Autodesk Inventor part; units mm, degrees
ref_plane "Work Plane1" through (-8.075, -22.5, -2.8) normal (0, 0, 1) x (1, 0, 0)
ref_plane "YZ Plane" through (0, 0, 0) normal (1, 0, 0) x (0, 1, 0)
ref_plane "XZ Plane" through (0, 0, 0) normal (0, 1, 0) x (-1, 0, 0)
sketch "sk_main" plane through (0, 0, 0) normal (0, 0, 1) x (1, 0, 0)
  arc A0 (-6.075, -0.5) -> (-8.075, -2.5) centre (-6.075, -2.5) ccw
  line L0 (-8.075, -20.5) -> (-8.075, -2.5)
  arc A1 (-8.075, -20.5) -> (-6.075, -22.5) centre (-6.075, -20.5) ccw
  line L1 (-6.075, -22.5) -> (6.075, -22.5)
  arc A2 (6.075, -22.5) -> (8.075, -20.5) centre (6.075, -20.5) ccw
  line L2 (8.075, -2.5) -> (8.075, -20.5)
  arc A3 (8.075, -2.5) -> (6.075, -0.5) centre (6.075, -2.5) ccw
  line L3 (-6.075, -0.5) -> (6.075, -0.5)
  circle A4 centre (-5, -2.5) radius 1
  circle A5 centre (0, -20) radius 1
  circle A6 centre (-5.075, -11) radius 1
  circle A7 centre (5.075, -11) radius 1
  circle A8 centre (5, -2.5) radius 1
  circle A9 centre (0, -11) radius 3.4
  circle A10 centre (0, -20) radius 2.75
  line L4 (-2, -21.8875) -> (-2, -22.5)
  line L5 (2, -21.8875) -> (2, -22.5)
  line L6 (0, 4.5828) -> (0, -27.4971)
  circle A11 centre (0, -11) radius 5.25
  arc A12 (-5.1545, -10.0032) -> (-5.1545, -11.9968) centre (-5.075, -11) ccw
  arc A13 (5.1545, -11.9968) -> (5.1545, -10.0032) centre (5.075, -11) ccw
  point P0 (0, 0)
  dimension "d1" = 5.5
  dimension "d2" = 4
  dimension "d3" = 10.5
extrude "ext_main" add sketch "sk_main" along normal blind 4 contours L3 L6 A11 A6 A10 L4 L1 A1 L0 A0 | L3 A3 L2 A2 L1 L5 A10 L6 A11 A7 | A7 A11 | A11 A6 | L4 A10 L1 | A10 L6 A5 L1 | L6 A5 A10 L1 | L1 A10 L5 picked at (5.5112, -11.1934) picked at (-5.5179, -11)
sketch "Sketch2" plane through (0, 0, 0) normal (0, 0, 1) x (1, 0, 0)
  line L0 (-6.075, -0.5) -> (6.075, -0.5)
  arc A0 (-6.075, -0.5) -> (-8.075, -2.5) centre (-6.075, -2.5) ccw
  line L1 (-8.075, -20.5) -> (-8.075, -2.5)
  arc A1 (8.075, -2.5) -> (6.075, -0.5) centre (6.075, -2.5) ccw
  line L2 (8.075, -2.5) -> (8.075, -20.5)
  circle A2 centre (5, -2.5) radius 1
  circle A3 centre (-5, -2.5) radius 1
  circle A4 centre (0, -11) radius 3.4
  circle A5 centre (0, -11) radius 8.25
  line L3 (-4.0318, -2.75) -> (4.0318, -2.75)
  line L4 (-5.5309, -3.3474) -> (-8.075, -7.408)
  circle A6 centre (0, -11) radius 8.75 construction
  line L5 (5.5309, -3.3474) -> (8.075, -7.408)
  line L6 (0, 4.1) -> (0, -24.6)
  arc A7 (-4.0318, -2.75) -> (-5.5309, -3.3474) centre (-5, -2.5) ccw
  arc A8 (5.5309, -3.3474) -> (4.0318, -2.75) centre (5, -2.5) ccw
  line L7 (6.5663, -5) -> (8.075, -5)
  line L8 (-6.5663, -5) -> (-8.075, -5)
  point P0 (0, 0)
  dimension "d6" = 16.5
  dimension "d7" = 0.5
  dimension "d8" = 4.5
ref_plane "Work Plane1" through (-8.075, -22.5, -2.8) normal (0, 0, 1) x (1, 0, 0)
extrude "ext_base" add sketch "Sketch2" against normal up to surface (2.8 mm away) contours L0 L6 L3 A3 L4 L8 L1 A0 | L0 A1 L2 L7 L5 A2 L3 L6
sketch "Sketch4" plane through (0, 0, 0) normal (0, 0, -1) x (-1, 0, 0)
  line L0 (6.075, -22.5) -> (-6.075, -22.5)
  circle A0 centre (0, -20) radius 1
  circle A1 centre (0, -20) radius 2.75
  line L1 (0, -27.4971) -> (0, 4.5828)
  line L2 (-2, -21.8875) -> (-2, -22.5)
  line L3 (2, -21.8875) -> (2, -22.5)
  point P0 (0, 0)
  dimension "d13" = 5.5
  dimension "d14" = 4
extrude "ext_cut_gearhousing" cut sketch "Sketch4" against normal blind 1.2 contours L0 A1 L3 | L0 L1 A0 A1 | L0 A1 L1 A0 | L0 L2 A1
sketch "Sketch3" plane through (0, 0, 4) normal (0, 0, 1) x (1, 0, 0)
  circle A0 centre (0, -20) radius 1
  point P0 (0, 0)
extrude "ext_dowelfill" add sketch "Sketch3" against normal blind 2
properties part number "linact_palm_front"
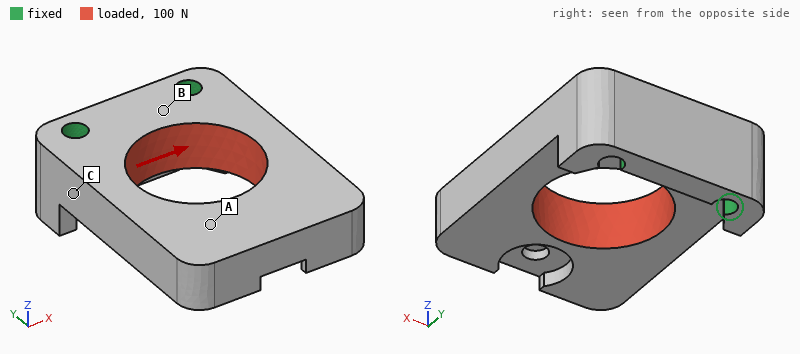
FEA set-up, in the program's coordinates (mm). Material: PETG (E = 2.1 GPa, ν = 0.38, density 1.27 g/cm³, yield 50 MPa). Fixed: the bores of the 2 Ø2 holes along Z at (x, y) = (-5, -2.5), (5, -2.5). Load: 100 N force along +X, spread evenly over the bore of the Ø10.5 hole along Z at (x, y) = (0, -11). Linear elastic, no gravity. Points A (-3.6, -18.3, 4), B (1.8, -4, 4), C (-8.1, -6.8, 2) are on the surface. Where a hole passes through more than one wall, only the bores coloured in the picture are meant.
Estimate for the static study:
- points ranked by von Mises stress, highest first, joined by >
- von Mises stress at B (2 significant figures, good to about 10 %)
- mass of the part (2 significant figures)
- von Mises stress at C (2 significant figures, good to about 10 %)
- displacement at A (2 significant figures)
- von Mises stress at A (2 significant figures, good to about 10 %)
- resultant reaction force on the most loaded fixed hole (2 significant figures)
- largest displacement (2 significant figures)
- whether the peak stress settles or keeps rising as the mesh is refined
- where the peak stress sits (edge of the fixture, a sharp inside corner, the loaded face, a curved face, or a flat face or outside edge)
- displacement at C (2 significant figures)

C > B > A
5.5 MPa
1.4 g
10 MPa
0.15 mm
1.6 MPa
78 N
0.17 mm
keeps rising
edge of the fixture
0.038 mm
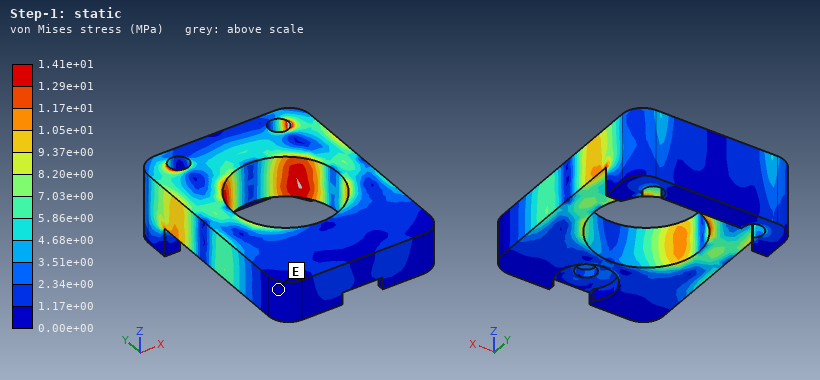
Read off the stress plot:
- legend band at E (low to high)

0.00e+00 to 1.17e+00 MPa
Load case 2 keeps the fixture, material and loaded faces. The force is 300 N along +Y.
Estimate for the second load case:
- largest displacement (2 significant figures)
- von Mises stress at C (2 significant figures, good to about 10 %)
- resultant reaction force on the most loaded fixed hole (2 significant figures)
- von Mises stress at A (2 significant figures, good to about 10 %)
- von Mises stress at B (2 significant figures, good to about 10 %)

79 µm
7.2 MPa
150 N
3.6 MPa
1.8 MPa
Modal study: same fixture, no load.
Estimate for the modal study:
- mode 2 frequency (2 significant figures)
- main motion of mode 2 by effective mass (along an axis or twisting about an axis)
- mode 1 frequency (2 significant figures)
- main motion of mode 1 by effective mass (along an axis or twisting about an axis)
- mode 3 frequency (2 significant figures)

3500 Hz
along X
1700 Hz
along Z
4000 Hz
